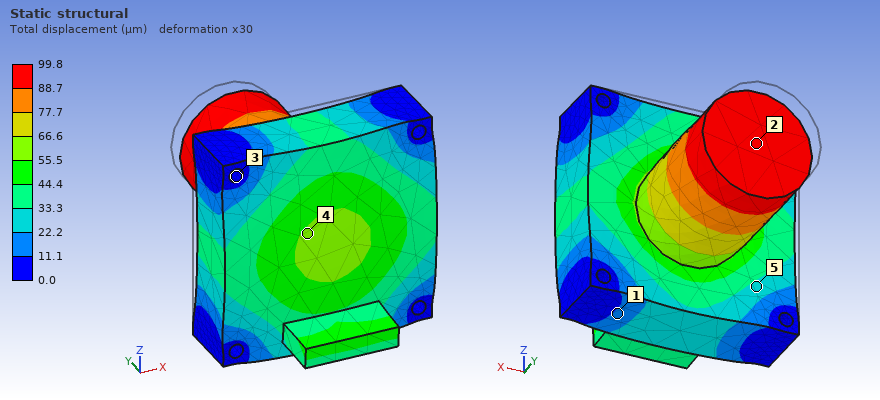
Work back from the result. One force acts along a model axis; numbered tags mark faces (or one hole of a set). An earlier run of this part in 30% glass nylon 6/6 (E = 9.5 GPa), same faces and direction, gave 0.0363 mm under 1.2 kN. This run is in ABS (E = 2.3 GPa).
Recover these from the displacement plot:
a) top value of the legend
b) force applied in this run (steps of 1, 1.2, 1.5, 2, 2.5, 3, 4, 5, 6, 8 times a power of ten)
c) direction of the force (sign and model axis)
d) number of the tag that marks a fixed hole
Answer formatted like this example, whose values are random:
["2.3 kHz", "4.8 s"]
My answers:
["99.8 µm", "800 N", "-Y", "3"]
